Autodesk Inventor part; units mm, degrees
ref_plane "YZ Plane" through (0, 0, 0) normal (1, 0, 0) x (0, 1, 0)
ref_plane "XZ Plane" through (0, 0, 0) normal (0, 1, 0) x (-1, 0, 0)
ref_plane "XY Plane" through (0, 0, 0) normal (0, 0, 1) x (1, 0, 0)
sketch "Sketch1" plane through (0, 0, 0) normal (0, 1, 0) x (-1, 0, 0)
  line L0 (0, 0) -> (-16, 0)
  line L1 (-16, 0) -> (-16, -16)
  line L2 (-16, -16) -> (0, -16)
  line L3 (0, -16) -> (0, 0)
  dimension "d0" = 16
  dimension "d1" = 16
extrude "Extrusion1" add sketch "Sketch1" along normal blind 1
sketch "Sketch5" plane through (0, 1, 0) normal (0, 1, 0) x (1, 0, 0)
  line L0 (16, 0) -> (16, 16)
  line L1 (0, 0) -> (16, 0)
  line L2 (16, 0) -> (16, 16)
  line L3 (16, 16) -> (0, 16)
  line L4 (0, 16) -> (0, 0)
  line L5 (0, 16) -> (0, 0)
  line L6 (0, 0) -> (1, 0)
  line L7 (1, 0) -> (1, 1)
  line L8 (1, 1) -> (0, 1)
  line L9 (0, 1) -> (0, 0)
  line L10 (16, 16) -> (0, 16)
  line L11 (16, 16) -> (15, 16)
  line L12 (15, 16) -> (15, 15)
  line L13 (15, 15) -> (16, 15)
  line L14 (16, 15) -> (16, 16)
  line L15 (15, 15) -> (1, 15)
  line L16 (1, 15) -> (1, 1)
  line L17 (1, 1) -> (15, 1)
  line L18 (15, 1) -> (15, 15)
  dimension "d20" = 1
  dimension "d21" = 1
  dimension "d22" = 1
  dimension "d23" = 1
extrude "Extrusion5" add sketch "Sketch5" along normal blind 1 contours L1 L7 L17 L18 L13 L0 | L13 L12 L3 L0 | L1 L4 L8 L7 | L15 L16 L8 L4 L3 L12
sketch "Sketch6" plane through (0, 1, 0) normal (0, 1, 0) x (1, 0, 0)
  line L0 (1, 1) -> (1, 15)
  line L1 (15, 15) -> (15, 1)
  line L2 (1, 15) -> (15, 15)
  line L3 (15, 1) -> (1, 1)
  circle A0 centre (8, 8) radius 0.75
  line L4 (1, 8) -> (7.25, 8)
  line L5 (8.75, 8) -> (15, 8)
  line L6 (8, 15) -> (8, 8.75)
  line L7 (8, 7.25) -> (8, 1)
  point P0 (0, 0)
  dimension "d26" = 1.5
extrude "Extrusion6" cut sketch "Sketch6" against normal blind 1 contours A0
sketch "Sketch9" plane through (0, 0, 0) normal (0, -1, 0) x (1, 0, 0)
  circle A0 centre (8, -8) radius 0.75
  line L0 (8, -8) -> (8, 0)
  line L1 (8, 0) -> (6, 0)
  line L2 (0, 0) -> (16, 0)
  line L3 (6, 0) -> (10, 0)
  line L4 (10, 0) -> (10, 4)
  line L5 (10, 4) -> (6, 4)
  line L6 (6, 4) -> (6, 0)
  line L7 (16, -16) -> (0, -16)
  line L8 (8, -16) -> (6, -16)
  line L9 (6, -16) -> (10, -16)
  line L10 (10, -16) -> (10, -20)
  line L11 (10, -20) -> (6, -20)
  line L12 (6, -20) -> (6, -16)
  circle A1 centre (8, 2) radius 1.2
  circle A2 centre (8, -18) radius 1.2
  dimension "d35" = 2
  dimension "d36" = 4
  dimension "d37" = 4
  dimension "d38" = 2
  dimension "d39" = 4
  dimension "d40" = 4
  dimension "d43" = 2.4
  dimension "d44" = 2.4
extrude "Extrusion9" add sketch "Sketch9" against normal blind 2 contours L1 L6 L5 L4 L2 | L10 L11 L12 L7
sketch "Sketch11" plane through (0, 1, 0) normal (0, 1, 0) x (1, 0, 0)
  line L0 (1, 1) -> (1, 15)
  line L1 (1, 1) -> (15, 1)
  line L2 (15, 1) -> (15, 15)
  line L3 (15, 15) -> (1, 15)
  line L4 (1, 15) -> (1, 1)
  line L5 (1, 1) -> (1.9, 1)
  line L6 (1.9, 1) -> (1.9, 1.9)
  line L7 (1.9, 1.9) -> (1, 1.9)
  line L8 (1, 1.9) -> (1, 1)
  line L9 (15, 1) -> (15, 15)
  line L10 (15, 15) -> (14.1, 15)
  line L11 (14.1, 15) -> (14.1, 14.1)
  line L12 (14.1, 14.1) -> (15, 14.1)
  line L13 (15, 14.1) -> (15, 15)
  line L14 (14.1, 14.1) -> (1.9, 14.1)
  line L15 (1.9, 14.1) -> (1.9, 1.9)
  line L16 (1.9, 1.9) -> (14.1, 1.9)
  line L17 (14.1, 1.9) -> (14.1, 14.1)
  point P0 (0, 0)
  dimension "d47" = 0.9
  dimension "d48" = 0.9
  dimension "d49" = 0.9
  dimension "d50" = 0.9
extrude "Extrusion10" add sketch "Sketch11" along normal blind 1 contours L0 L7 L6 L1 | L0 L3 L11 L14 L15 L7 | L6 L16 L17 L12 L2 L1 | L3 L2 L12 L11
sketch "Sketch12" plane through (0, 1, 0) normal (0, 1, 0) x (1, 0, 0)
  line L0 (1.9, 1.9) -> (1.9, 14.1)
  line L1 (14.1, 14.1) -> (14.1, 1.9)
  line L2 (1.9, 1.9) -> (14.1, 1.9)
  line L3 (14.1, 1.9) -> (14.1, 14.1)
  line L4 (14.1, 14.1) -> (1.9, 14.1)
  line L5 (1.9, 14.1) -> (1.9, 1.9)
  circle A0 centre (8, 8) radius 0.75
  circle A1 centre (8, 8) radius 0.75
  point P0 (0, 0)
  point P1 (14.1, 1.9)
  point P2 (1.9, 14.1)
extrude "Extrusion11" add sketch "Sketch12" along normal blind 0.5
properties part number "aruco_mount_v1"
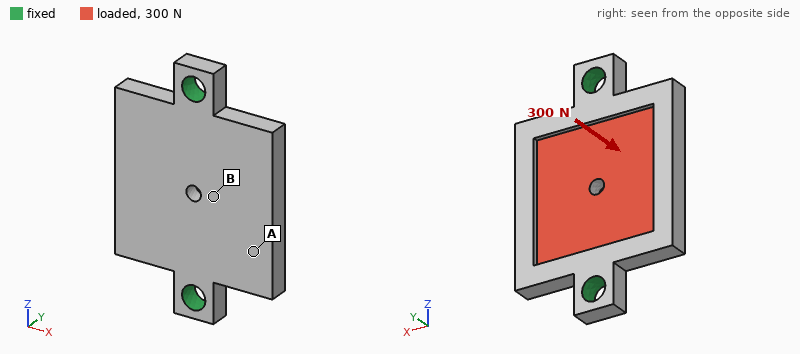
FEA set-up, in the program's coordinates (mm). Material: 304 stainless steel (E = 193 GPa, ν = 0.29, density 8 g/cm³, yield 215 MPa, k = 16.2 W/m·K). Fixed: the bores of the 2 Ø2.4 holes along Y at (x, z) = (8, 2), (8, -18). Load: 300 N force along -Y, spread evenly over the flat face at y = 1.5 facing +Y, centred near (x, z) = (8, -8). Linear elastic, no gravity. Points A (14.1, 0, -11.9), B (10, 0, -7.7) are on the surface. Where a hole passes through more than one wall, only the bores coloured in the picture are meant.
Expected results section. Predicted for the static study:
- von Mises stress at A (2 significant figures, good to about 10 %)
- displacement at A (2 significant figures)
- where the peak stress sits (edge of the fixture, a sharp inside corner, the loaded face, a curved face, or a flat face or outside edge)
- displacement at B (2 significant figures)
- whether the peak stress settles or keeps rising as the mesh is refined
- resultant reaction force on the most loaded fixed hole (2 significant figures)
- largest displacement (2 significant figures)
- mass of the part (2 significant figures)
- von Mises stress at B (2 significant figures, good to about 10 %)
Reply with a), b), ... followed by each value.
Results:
a) 34 MPa
b) 9.7 µm
c) edge of the fixture
d) 10 µm
e) keeps rising
f) 170 N
g) 13 µm
h) 3.8 g
i) 68 MPa
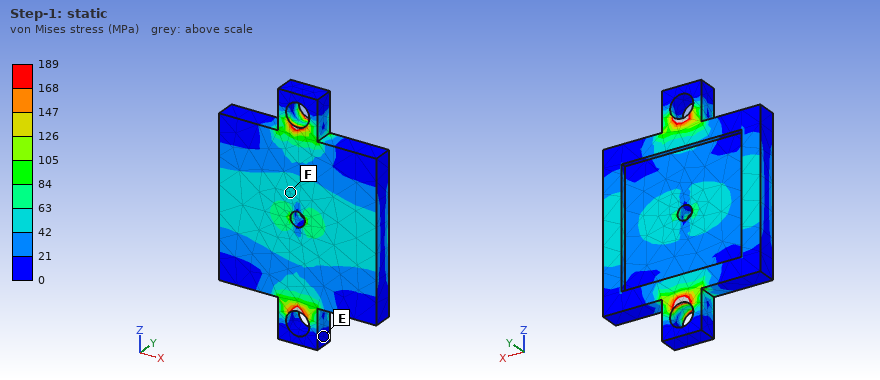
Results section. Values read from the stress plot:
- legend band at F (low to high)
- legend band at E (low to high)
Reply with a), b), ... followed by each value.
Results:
a) 42 to 63 MPa
b) 0 to 21 MPa
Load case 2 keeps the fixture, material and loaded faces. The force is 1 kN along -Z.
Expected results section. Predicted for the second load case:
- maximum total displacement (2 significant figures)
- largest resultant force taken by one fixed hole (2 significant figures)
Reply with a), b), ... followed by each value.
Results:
a) 2.9 µm
b) 500 N
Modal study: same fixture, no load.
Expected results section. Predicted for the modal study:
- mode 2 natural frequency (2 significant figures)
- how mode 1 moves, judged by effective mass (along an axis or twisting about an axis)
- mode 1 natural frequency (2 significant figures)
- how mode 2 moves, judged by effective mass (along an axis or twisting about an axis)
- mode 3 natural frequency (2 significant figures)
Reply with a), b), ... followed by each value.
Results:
a) 15 kHz
b) twisting about Z
c) 11 kHz
d) along Y
e) 27 kHz
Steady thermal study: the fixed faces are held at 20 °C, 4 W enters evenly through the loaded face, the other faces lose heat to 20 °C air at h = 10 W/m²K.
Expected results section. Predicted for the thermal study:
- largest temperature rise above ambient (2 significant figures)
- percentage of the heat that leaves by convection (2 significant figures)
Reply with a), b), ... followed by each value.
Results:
a) 59 K
b) 6.1 %
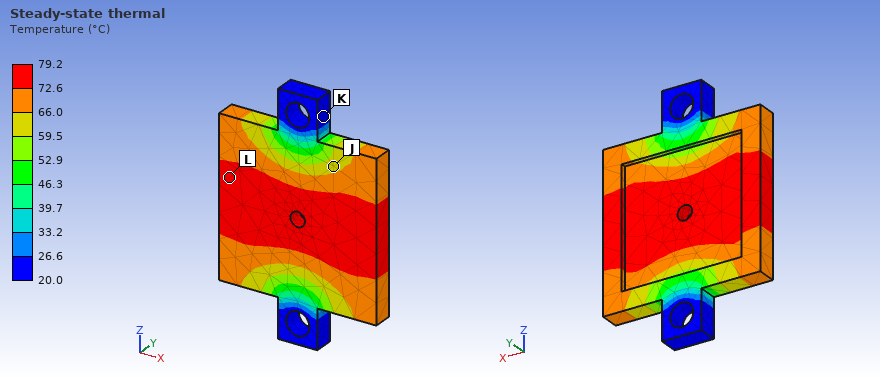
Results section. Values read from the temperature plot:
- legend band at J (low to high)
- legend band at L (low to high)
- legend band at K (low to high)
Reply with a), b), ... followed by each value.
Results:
a) 59.5 to 66.0 °C
b) 72.6 to 79.2 °C
c) 20.0 to 26.6 °C
